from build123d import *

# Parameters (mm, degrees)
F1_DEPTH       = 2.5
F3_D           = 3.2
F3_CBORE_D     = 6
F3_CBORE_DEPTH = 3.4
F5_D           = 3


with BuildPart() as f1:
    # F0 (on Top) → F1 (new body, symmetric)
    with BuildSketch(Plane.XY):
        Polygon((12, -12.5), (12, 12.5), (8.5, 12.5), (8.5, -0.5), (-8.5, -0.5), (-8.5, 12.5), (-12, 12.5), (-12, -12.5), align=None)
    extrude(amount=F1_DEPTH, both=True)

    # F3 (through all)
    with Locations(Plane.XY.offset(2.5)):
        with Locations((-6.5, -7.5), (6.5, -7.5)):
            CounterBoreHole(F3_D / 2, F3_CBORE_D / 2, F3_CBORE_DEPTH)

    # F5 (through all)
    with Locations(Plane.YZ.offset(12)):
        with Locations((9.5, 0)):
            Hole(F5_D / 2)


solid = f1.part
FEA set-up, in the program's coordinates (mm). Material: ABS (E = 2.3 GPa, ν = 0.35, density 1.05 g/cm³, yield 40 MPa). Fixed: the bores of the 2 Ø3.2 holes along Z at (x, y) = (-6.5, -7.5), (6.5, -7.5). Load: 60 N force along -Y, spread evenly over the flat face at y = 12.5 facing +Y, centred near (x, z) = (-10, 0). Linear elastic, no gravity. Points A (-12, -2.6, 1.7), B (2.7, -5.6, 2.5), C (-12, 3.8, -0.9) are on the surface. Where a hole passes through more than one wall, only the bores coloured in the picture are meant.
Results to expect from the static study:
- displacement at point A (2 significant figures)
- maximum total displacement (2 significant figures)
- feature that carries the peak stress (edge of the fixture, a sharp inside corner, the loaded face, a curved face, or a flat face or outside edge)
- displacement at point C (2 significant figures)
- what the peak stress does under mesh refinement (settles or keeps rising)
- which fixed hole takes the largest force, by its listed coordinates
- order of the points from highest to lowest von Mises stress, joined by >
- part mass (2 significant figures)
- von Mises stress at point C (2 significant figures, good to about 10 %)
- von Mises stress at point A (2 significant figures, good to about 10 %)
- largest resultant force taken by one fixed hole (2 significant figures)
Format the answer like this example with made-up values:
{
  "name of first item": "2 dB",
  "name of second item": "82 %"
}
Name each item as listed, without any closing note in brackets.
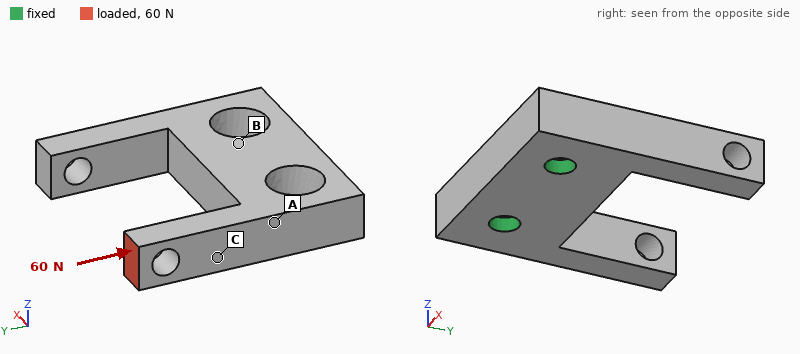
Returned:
{
  "displacement at point A": "0.049 mm",
  "maximum total displacement": "0.14 mm",
  "feature that carries the peak stress": "edge of the fixture",
  "displacement at point C": "0.078 mm",
  "what the peak stress does under mesh refinement": "keeps rising",
  "which fixed hole takes the largest force, by its listed coordinates": "(-6.5, -7.5)",
  "order of the points from highest to lowest von Mises stress, joined by >": "A > C > B",
  "part mass": "1.7 g",
  "von Mises stress at point C": "3.2 MPa",
  "von Mises stress at point A": "4.5 MPa",
  "largest resultant force taken by one fixed hole": "70 N"
}
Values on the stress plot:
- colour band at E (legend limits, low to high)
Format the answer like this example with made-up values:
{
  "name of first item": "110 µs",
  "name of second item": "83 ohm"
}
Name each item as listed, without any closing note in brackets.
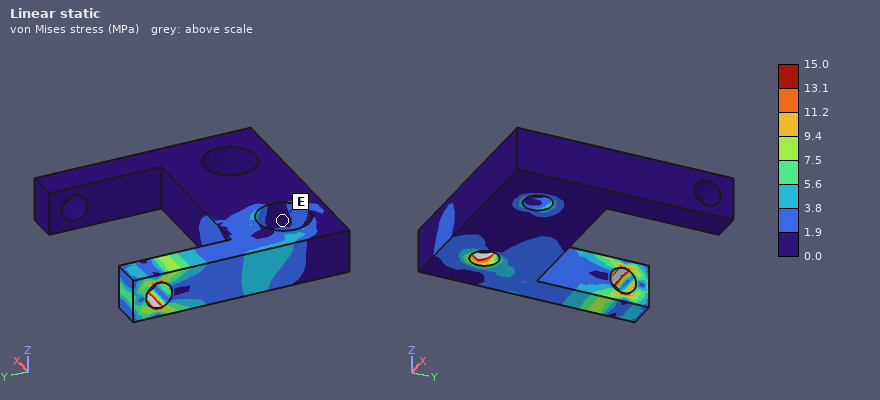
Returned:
{
  "colour band at E": "0.0 to 1.9 MPa"
}
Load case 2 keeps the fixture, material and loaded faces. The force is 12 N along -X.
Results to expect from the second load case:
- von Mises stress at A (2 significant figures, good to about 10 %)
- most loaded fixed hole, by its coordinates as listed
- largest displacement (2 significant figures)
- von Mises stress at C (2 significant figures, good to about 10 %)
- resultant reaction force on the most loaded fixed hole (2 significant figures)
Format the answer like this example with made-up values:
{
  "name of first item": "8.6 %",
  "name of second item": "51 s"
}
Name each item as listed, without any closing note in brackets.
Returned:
{
  "von Mises stress at A": "7.9 MPa",
  "most loaded fixed hole, by its coordinates as listed": "(6.5, -7.5)",
  "largest displacement": "0.40 mm",
  "von Mises stress at C": "10 MPa",
  "resultant reaction force on the most loaded fixed hole": "18 N"
}
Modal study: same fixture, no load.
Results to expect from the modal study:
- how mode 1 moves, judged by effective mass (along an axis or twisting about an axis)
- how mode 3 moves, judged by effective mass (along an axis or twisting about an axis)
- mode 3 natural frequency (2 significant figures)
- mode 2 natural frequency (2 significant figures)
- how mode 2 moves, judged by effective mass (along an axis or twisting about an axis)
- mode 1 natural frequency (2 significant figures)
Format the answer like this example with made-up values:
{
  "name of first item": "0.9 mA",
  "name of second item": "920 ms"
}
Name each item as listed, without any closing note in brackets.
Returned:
{
  "how mode 1 moves, judged by effective mass": "along Z",
  "how mode 3 moves, judged by effective mass": "along X",
  "mode 3 natural frequency": "3700 Hz",
  "mode 2 natural frequency": "3100 Hz",
  "how mode 2 moves, judged by effective mass": "twisting about Y",
  "mode 1 natural frequency": "2500 Hz"
}
